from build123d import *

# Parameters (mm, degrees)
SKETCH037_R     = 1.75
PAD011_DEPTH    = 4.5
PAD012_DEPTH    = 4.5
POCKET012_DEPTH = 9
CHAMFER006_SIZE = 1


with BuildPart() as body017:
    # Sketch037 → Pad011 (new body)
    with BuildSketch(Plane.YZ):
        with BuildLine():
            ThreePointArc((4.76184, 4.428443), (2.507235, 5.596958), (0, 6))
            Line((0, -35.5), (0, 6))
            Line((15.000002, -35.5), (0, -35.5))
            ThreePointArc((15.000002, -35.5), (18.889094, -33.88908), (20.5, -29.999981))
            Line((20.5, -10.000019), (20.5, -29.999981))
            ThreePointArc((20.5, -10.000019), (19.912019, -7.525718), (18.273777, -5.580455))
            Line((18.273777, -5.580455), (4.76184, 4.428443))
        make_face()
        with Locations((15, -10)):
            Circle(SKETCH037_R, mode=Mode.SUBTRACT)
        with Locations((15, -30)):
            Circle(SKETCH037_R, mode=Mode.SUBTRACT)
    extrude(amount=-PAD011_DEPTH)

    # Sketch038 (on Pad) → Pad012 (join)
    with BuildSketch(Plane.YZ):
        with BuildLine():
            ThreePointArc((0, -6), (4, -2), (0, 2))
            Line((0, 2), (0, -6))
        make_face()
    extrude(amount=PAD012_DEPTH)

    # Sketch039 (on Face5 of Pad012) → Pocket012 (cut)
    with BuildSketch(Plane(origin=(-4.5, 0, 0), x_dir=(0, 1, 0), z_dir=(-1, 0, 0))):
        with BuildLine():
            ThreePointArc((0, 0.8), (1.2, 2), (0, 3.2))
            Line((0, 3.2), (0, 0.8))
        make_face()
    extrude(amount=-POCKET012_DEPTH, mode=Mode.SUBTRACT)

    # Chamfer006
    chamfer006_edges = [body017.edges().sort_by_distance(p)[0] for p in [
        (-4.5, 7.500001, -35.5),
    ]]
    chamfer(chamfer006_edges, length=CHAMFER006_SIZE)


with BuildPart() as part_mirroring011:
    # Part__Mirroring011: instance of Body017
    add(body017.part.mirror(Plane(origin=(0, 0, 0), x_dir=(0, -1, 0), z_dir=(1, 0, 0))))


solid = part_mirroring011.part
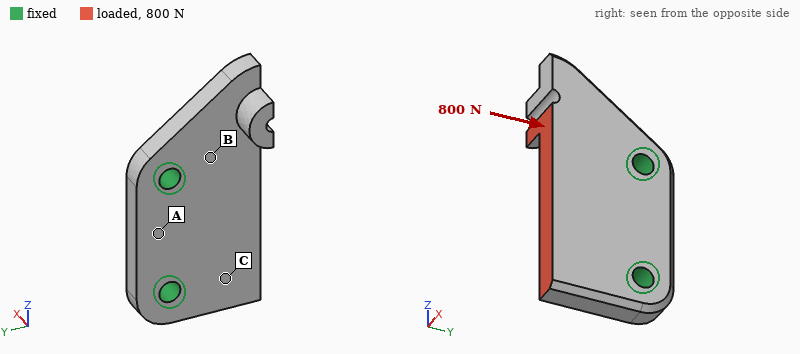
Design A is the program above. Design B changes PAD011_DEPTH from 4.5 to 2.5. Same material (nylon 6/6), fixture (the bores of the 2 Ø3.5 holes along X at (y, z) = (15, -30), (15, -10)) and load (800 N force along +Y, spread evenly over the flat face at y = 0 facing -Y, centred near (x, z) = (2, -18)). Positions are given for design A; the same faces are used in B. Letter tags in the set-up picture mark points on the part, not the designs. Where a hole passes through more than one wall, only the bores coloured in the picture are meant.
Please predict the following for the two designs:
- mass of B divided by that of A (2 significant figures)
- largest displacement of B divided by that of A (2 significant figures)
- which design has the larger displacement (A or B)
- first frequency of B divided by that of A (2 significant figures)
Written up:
0.56
4.1
B
0.57
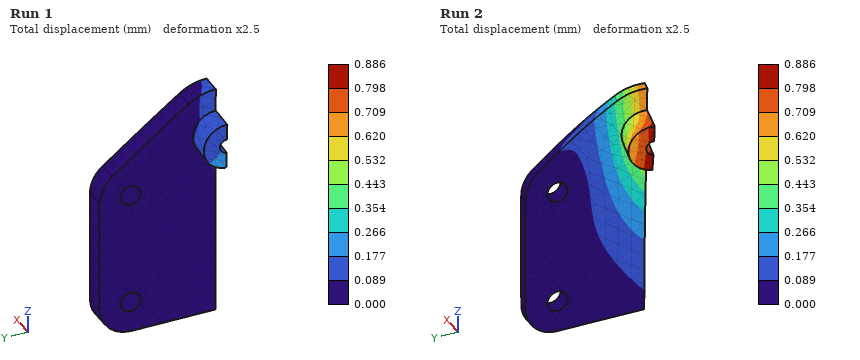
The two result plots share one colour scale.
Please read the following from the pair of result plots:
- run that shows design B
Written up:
Run 2
